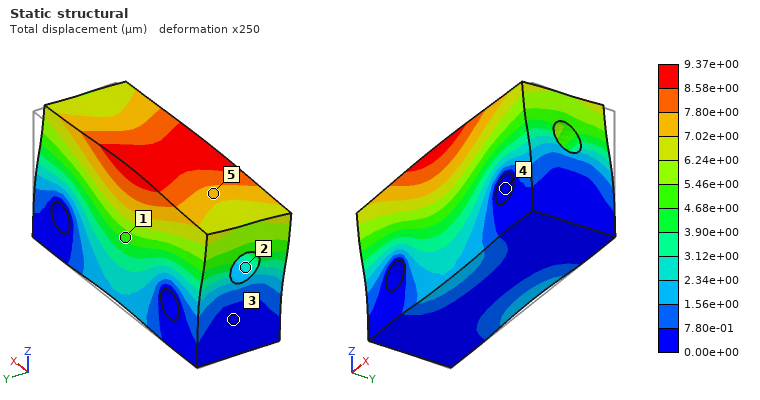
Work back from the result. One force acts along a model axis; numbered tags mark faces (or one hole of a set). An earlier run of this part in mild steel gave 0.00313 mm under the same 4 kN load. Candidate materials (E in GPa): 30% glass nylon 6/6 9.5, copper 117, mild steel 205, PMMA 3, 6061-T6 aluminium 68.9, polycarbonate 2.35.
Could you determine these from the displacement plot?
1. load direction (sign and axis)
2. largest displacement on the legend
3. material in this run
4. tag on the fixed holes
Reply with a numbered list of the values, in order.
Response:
1. -Y
2. 9.37e+00 µm
3. 6061-T6 aluminium
4. 4
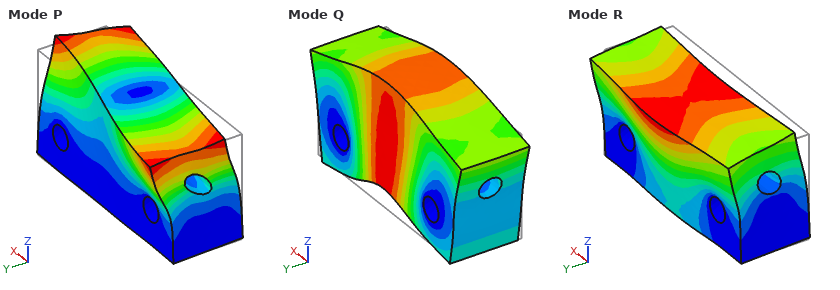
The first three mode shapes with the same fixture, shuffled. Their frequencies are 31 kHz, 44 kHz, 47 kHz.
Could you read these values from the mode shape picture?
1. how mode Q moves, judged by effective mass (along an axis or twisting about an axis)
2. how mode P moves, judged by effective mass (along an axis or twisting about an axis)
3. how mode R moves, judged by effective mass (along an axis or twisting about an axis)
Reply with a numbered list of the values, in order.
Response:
1. along Z
2. twisting about Z
3. along Y
